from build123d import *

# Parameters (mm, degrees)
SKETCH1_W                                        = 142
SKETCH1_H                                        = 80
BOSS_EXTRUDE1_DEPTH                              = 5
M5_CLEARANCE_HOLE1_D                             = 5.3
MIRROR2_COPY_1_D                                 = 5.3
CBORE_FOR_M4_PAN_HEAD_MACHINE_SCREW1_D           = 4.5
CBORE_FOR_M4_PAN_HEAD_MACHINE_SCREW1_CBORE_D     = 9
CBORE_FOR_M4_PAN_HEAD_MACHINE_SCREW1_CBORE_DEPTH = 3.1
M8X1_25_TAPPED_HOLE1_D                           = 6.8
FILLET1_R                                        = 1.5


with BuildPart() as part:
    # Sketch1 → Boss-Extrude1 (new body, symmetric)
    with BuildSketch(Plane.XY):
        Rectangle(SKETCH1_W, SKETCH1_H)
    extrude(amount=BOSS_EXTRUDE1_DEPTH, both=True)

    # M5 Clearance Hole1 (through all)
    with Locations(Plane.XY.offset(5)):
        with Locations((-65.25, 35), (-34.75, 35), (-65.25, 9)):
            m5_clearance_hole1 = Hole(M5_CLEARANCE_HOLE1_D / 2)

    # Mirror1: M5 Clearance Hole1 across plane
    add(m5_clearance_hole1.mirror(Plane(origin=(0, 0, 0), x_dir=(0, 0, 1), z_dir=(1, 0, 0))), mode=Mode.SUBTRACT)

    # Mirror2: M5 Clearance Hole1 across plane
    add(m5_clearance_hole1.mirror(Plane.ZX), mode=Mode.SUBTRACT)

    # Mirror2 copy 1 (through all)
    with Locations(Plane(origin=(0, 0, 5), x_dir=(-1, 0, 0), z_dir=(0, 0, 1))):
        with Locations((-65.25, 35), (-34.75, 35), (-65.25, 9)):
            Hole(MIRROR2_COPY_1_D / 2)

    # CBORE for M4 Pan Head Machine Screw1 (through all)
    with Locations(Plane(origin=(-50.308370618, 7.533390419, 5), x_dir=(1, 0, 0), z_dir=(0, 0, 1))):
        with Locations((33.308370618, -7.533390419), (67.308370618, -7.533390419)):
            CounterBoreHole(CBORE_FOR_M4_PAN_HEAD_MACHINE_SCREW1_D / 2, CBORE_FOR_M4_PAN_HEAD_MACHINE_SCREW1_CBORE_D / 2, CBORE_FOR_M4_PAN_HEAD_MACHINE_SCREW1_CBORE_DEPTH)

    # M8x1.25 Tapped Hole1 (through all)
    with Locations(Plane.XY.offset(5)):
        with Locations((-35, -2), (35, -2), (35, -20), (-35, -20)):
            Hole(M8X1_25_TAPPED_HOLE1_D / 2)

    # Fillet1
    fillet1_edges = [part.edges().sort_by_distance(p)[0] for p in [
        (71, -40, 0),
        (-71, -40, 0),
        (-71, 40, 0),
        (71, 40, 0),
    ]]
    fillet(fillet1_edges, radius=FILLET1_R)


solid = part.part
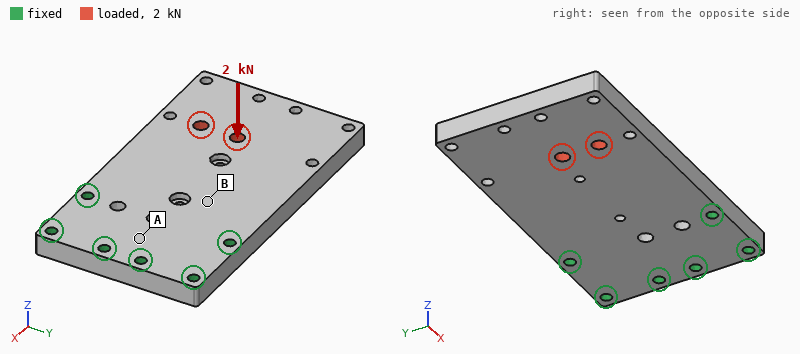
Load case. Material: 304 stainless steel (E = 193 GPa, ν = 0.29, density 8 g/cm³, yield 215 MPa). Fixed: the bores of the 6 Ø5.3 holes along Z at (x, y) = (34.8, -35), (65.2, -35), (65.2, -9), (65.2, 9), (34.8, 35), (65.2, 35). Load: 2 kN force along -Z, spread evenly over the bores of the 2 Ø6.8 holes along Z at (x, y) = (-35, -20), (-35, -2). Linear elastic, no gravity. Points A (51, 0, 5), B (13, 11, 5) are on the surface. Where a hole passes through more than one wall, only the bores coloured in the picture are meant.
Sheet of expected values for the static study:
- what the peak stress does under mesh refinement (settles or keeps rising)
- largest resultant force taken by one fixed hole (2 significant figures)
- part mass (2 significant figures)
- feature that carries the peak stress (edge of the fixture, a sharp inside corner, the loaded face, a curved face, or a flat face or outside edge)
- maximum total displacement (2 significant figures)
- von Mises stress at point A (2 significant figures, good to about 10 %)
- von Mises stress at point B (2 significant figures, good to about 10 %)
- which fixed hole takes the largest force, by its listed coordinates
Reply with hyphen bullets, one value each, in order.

- keeps rising
- 2.3 kN
- 870 g
- edge of the fixture
- 0.41 mm
- 23 MPa
- 72 MPa
- (34.8, -35)
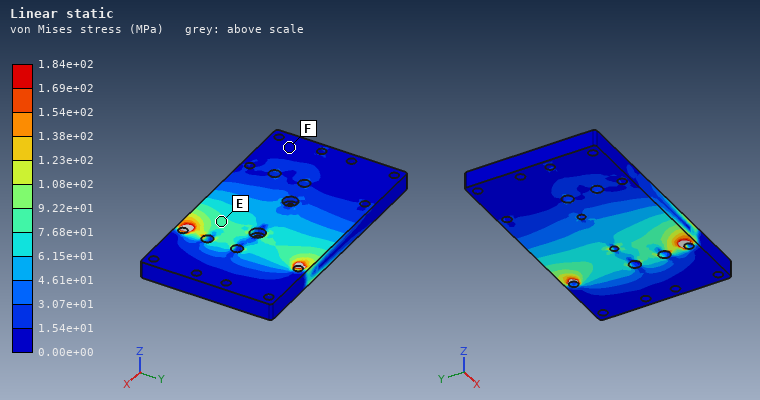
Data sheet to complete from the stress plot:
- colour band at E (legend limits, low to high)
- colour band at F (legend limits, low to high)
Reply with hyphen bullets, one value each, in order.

- 7.68e+01 to 9.22e+01 MPa
- 0.00e+00 to 1.54e+01 MPa
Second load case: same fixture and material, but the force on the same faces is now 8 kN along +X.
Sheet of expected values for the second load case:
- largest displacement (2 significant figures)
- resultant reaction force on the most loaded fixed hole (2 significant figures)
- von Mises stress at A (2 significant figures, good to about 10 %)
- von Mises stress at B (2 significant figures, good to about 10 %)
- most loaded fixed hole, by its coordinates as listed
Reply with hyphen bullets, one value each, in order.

- 8.6 µm
- 3.7 kN
- 5.6 MPa
- 7.9 MPa
- (34.8, -35)
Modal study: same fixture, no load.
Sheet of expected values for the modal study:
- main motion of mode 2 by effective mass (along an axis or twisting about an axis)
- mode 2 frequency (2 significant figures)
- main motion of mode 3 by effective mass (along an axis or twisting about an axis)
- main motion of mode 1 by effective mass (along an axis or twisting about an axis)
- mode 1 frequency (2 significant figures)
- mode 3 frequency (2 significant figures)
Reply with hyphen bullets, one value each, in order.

- twisting about X
- 2100 Hz
- along Z
- along Z
- 650 Hz
- 3800 Hz
